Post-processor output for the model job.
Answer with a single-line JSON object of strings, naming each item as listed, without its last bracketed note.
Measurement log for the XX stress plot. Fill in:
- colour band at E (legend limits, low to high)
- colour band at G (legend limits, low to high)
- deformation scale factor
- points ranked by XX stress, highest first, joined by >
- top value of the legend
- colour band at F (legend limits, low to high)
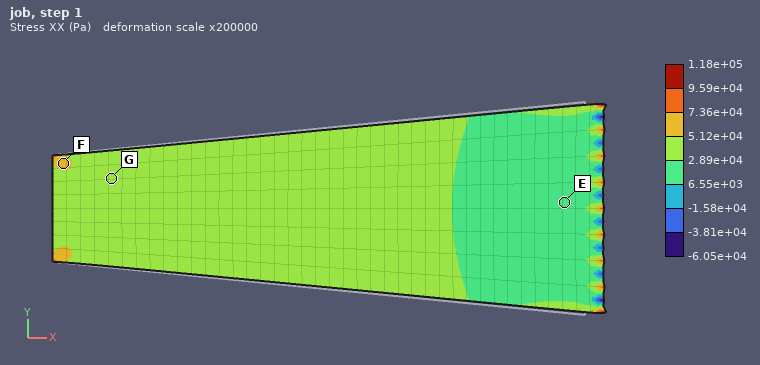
{"colour band at E": "6.55e+03 to 2.89e+04 Pa", "colour band at G": "2.89e+04 to 5.12e+04 Pa", "deformation scale factor": "200000", "points ranked by XX stress, highest first, joined by >": "F > G > E", "top value of the legend": "1.18e+05 Pa", "colour band at F": "5.12e+04 to 7.36e+04 Pa"}
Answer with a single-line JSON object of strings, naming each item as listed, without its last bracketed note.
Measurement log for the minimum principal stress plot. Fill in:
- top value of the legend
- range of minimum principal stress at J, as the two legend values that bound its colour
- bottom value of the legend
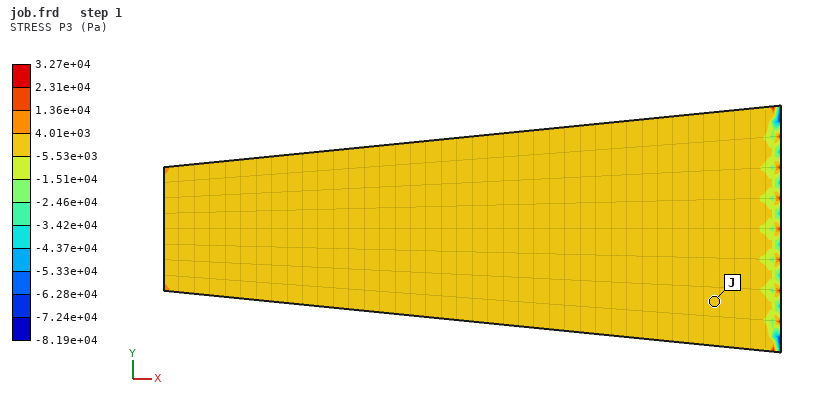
{"top value of the legend": "3.27e+04 Pa", "range of minimum principal stress at J, as the two legend values that bound its colour": "-5.53e+03 to 4.01e+03 Pa", "bottom value of the legend": "-8.19e+04 Pa"}
